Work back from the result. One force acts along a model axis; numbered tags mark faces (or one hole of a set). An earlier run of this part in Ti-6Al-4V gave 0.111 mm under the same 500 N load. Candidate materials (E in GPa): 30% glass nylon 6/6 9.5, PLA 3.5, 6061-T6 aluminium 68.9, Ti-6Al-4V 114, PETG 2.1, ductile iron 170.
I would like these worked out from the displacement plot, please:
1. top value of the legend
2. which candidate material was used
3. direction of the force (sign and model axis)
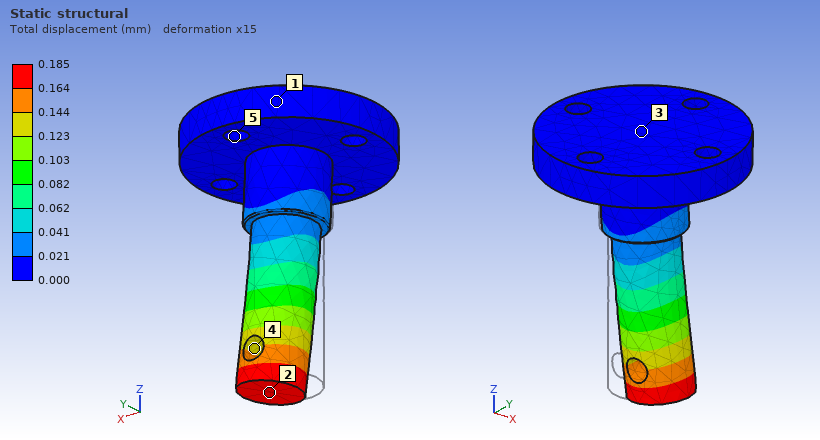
0.185 mm
6061-T6 aluminium
+X
